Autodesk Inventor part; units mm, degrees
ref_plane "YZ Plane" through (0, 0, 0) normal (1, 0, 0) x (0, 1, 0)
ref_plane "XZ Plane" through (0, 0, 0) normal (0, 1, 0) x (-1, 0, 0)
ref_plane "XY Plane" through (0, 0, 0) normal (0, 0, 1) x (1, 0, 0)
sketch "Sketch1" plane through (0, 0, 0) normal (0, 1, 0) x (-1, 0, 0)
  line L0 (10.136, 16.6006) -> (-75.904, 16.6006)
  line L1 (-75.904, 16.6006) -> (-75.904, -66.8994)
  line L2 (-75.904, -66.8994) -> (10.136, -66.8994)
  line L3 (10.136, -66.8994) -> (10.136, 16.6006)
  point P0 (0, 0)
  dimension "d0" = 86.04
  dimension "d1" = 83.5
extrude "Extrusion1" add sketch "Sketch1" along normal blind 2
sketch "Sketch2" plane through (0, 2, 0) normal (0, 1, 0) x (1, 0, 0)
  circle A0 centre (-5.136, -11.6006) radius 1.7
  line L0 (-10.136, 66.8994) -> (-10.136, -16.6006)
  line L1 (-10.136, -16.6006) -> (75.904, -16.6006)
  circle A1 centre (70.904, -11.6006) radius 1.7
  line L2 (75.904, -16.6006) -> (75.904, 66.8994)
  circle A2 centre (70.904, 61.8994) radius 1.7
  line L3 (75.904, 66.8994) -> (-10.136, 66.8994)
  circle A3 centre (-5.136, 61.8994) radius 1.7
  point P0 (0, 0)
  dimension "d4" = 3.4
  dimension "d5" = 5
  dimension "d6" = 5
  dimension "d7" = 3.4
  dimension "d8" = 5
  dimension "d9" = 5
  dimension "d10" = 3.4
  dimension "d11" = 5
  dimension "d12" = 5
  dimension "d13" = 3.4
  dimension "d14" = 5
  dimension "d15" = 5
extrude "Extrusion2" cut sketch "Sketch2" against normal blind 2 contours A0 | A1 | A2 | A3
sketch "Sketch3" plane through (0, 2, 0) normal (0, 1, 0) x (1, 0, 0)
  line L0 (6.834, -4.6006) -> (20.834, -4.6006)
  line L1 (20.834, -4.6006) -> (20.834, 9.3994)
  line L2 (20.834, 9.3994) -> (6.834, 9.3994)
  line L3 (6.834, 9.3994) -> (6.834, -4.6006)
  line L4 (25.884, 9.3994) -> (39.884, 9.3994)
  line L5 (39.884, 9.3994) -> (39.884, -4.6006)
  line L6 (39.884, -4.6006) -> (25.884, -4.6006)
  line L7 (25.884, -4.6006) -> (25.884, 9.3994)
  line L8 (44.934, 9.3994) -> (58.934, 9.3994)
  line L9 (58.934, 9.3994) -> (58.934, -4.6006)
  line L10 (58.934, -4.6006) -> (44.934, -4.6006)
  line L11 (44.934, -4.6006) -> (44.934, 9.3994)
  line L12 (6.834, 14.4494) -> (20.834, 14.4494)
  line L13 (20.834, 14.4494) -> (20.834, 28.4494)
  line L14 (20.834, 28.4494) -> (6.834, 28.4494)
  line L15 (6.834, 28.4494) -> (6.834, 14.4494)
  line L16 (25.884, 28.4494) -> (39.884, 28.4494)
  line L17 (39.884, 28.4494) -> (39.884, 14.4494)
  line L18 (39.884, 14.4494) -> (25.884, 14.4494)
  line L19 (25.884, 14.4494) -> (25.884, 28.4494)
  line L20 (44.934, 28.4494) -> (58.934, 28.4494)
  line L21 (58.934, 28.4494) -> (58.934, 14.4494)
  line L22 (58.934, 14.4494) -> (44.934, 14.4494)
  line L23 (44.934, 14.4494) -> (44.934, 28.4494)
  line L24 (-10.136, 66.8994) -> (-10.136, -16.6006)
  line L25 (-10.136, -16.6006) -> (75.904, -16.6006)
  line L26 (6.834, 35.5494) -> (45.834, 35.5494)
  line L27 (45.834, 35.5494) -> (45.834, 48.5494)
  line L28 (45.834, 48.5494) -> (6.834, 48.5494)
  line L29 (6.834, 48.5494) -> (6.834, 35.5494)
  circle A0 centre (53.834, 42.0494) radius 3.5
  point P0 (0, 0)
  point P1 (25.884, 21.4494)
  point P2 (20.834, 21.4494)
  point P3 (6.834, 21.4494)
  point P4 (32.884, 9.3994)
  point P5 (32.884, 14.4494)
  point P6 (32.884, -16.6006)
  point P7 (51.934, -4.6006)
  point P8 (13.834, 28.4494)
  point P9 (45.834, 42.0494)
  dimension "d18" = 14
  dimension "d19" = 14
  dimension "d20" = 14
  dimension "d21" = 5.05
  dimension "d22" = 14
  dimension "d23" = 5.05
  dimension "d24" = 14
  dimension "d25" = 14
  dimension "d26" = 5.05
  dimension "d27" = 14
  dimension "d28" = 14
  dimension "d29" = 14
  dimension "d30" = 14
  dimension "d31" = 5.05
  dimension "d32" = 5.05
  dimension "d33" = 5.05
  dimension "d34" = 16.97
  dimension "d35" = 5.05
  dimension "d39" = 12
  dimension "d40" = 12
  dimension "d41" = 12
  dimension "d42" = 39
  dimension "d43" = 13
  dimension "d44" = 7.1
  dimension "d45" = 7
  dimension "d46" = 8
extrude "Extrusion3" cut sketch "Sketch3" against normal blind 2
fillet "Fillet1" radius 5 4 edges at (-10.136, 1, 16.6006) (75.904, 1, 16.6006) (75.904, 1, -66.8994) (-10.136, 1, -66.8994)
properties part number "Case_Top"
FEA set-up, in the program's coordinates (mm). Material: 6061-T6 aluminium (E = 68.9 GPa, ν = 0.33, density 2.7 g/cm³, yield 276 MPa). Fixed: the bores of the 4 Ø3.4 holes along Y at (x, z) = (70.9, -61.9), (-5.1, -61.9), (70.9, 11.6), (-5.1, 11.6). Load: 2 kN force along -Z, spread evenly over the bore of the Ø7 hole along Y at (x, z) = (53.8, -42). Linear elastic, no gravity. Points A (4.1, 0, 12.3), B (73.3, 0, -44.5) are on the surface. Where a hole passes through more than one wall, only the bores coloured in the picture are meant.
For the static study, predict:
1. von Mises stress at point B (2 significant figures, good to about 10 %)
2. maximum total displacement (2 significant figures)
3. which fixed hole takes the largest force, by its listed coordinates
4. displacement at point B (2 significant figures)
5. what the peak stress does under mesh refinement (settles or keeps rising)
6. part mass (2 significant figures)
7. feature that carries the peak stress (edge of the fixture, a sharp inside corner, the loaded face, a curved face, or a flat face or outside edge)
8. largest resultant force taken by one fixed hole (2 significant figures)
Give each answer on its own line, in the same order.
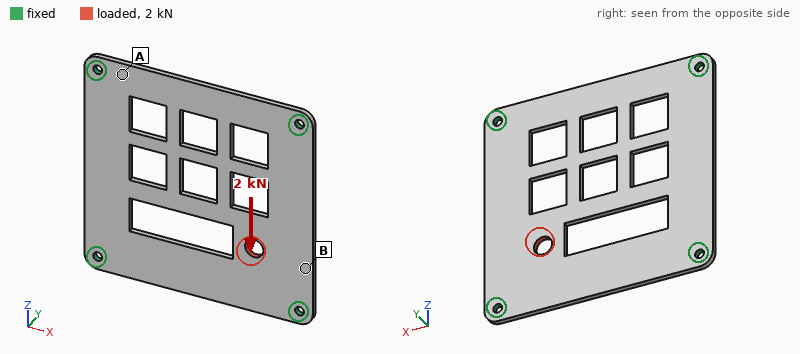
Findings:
16 MPa
31 µm
(70.9, -61.9)
9.4 µm
keeps rising
29 g
edge of the fixture
1.2 kN
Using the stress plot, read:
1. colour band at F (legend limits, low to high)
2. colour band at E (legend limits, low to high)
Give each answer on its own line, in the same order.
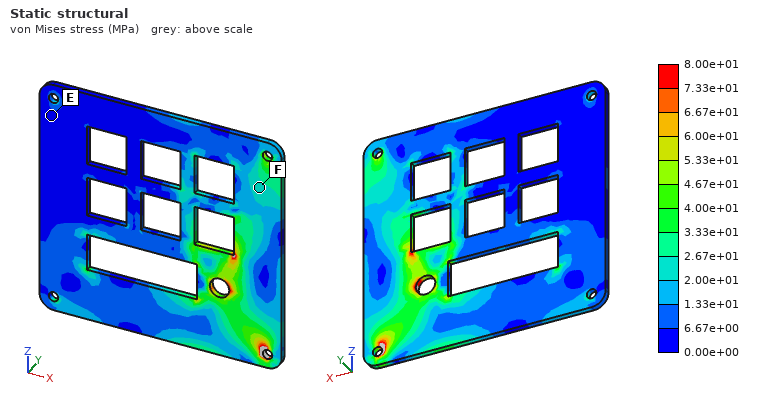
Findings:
2.00e+01 to 2.67e+01 MPa
0.00e+00 to 6.67e+00 MPa
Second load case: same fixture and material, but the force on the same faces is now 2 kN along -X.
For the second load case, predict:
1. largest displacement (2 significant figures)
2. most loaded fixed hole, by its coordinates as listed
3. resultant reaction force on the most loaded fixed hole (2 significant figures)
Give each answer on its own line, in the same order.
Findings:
39 µm
(70.9, -61.9)
1.1 kN
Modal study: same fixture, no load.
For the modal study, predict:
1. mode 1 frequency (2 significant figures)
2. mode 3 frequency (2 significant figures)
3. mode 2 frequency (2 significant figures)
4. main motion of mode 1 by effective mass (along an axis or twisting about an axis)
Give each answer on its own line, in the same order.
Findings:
1200 Hz
2000 Hz
2000 Hz
along Y
